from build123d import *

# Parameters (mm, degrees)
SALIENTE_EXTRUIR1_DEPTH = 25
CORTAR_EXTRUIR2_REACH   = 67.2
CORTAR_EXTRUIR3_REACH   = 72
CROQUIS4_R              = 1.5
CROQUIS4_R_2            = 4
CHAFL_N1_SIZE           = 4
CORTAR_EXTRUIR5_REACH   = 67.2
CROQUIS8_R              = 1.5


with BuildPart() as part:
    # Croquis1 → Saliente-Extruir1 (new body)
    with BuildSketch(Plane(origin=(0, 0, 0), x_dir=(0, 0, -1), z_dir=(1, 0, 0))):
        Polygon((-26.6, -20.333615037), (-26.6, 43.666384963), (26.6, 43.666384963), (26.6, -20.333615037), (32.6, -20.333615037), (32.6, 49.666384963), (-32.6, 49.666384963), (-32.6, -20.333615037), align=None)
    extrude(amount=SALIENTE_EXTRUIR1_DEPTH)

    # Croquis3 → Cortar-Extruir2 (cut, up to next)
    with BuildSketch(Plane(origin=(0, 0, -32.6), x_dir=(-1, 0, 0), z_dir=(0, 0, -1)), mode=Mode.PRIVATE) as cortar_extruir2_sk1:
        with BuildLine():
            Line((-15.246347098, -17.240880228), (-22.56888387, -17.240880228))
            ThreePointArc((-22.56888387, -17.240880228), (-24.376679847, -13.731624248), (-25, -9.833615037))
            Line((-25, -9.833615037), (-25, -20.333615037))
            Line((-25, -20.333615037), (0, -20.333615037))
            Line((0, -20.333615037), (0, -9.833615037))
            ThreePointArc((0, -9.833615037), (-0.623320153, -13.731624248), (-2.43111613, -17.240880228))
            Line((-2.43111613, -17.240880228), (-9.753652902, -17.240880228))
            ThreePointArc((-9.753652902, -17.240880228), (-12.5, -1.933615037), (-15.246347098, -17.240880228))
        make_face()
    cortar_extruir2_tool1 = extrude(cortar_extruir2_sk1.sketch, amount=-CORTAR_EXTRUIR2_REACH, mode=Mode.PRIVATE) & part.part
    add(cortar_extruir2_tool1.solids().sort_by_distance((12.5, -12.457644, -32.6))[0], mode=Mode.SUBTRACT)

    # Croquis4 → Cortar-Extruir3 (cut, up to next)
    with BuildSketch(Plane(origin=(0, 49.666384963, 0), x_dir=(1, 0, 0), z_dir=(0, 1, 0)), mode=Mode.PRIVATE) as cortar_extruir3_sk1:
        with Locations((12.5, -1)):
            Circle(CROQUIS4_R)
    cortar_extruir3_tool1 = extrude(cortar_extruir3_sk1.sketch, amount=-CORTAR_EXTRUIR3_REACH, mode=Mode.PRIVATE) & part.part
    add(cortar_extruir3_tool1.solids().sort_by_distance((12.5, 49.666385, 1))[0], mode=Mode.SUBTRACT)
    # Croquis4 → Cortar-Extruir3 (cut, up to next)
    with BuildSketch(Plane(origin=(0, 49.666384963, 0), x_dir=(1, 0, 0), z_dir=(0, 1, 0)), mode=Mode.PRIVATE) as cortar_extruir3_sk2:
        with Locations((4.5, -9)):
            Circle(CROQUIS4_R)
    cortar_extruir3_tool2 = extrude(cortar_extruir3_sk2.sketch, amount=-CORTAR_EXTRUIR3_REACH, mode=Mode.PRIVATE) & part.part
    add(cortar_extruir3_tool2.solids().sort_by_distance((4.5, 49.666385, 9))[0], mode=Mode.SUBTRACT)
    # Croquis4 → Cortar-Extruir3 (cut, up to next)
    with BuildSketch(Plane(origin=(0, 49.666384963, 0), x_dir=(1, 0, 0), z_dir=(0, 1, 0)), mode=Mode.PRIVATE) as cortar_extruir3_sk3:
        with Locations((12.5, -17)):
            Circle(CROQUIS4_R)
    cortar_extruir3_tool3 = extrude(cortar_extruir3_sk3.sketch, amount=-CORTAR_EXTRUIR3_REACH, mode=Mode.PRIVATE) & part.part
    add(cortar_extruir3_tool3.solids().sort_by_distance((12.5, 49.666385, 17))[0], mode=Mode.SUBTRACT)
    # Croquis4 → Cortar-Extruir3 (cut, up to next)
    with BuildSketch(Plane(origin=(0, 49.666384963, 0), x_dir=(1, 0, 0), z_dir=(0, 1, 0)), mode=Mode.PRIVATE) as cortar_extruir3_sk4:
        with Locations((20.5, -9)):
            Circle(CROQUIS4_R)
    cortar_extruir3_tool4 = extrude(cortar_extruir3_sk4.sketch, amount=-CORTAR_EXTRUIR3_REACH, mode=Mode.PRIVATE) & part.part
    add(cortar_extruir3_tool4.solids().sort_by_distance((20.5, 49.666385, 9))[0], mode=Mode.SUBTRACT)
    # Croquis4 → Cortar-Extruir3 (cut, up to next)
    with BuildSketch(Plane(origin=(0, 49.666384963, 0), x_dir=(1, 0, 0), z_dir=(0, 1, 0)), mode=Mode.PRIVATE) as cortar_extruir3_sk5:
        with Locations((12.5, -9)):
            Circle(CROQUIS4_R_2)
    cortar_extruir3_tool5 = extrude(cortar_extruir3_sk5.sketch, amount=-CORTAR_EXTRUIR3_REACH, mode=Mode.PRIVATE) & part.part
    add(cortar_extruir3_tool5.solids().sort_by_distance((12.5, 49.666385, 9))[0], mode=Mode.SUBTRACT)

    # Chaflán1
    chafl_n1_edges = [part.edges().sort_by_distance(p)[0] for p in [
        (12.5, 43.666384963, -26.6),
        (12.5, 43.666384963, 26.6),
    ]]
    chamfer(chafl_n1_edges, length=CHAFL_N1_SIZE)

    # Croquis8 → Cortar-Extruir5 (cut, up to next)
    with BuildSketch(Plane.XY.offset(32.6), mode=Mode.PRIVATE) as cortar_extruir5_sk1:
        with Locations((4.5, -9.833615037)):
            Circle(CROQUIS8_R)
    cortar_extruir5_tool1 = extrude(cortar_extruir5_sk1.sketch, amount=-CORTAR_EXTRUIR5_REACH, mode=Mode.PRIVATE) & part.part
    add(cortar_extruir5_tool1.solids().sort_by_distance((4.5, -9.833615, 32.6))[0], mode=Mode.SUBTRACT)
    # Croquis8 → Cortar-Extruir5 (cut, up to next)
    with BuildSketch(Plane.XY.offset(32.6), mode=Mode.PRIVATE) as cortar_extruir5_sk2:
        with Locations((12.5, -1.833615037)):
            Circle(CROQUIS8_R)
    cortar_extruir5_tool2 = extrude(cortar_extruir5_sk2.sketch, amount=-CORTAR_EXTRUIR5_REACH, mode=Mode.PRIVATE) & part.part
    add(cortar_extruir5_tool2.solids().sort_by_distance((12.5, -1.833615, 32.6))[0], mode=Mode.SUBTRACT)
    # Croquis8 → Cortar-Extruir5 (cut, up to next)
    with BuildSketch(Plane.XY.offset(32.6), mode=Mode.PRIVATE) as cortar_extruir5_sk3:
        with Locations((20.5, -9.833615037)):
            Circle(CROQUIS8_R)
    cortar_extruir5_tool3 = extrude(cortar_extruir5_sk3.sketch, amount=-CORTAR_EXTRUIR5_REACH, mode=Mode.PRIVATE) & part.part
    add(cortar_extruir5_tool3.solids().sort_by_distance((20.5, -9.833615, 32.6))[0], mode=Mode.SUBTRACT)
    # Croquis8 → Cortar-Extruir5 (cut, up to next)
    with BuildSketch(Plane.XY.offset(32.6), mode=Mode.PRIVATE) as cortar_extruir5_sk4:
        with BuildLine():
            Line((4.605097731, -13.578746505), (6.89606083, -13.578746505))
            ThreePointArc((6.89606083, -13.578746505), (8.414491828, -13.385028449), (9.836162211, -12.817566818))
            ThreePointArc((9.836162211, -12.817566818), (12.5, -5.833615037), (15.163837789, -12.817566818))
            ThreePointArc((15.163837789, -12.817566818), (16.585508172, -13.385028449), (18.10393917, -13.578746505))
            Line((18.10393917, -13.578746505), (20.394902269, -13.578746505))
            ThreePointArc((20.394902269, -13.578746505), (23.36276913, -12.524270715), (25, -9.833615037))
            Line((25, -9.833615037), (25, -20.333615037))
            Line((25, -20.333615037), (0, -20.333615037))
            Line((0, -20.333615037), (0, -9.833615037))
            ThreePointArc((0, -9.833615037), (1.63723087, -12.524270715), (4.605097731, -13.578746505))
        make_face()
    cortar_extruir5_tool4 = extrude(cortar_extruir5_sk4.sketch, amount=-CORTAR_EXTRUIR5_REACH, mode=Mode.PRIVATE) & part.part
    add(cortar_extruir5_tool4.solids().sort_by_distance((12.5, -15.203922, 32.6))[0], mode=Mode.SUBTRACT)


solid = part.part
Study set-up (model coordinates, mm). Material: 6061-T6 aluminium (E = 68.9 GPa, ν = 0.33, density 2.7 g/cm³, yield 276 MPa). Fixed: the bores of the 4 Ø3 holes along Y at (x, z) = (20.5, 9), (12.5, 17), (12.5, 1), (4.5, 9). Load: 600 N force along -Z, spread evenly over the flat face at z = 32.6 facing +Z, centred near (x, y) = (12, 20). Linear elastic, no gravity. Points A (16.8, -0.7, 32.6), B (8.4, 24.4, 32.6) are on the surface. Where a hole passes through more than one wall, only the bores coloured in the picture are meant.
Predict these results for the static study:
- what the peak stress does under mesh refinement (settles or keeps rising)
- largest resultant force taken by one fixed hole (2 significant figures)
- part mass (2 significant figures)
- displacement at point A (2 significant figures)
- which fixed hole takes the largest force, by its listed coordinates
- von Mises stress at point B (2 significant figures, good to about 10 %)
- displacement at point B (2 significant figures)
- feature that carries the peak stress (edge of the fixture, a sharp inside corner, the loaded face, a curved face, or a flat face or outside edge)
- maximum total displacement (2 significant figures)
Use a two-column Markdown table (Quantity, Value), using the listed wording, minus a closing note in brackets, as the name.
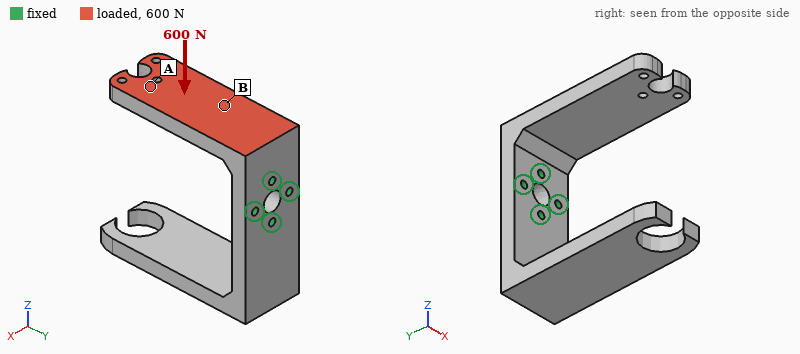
| Quantity | Value |
|---|---|
| what the peak stress does under mesh refinement | keeps rising |
| largest resultant force taken by one fixed hole | 930 N |
| part mass | 69 g |
| displacement at point A | 0.49 mm |
| which fixed hole takes the largest force, by its listed coordinates | (12.5, 17) |
| von Mises stress at point B | 39 MPa |
| displacement at point B | 0.19 mm |
| feature that carries the peak stress | edge of the fixture |
| maximum total displacement | 0.66 mm |
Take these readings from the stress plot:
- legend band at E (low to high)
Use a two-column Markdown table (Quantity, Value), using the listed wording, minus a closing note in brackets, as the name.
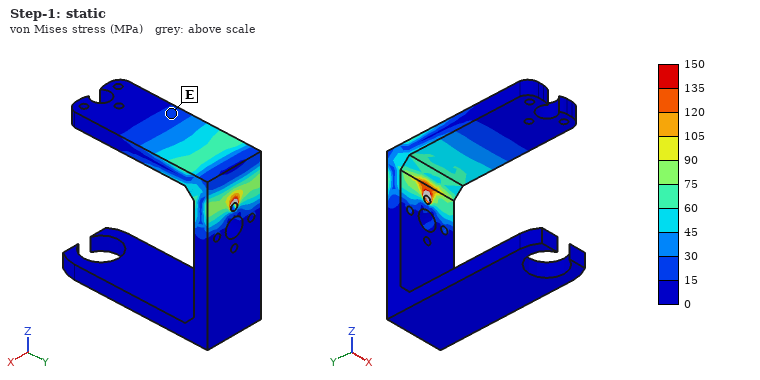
| Quantity | Value |
|---|---|
| legend band at E | 15 to 30 MPa |
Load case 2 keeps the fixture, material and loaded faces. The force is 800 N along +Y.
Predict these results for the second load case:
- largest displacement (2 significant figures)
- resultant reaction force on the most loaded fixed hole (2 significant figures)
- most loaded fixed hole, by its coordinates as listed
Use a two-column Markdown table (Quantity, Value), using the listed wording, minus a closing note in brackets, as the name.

| Quantity | Value |
|---|---|
| largest displacement | 0.26 mm |
| resultant reaction force on the most loaded fixed hole | 1.2 kN |
| most loaded fixed hole, by its coordinates as listed | (12.5, 17) |
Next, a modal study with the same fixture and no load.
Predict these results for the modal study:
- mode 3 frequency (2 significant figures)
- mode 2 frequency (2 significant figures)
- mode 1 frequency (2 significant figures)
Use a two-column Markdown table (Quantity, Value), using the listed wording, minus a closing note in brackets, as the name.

| Quantity | Value |
|---|---|
| mode 3 frequency | 1200 Hz |
| mode 2 frequency | 1200 Hz |
| mode 1 frequency | 850 Hz |
